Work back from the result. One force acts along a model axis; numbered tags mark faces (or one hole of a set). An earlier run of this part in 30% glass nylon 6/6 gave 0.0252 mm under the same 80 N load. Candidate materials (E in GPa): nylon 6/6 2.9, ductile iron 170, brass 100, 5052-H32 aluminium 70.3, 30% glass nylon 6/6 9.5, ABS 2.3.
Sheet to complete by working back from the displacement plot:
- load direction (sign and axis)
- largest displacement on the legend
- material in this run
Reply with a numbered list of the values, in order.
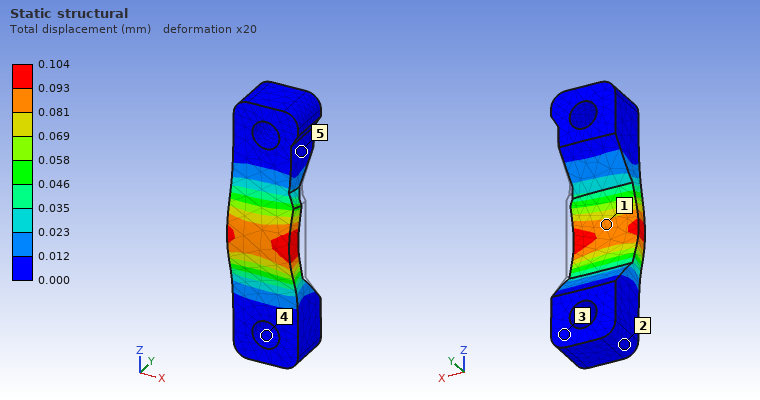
1. -Y
2. 0.104 mm
3. ABS
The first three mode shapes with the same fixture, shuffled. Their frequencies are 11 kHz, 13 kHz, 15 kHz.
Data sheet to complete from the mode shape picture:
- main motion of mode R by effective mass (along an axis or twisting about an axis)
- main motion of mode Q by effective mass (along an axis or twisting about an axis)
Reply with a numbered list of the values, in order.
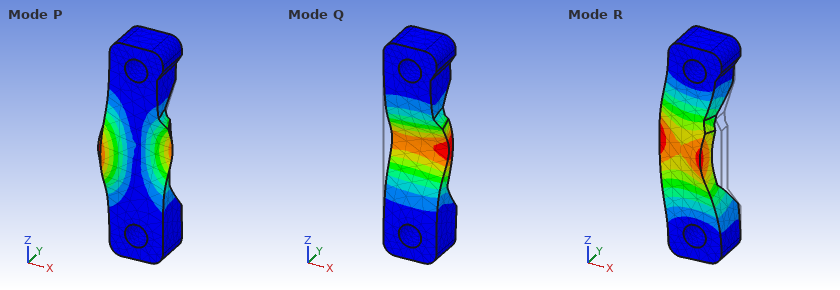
1. along X
2. along Y
